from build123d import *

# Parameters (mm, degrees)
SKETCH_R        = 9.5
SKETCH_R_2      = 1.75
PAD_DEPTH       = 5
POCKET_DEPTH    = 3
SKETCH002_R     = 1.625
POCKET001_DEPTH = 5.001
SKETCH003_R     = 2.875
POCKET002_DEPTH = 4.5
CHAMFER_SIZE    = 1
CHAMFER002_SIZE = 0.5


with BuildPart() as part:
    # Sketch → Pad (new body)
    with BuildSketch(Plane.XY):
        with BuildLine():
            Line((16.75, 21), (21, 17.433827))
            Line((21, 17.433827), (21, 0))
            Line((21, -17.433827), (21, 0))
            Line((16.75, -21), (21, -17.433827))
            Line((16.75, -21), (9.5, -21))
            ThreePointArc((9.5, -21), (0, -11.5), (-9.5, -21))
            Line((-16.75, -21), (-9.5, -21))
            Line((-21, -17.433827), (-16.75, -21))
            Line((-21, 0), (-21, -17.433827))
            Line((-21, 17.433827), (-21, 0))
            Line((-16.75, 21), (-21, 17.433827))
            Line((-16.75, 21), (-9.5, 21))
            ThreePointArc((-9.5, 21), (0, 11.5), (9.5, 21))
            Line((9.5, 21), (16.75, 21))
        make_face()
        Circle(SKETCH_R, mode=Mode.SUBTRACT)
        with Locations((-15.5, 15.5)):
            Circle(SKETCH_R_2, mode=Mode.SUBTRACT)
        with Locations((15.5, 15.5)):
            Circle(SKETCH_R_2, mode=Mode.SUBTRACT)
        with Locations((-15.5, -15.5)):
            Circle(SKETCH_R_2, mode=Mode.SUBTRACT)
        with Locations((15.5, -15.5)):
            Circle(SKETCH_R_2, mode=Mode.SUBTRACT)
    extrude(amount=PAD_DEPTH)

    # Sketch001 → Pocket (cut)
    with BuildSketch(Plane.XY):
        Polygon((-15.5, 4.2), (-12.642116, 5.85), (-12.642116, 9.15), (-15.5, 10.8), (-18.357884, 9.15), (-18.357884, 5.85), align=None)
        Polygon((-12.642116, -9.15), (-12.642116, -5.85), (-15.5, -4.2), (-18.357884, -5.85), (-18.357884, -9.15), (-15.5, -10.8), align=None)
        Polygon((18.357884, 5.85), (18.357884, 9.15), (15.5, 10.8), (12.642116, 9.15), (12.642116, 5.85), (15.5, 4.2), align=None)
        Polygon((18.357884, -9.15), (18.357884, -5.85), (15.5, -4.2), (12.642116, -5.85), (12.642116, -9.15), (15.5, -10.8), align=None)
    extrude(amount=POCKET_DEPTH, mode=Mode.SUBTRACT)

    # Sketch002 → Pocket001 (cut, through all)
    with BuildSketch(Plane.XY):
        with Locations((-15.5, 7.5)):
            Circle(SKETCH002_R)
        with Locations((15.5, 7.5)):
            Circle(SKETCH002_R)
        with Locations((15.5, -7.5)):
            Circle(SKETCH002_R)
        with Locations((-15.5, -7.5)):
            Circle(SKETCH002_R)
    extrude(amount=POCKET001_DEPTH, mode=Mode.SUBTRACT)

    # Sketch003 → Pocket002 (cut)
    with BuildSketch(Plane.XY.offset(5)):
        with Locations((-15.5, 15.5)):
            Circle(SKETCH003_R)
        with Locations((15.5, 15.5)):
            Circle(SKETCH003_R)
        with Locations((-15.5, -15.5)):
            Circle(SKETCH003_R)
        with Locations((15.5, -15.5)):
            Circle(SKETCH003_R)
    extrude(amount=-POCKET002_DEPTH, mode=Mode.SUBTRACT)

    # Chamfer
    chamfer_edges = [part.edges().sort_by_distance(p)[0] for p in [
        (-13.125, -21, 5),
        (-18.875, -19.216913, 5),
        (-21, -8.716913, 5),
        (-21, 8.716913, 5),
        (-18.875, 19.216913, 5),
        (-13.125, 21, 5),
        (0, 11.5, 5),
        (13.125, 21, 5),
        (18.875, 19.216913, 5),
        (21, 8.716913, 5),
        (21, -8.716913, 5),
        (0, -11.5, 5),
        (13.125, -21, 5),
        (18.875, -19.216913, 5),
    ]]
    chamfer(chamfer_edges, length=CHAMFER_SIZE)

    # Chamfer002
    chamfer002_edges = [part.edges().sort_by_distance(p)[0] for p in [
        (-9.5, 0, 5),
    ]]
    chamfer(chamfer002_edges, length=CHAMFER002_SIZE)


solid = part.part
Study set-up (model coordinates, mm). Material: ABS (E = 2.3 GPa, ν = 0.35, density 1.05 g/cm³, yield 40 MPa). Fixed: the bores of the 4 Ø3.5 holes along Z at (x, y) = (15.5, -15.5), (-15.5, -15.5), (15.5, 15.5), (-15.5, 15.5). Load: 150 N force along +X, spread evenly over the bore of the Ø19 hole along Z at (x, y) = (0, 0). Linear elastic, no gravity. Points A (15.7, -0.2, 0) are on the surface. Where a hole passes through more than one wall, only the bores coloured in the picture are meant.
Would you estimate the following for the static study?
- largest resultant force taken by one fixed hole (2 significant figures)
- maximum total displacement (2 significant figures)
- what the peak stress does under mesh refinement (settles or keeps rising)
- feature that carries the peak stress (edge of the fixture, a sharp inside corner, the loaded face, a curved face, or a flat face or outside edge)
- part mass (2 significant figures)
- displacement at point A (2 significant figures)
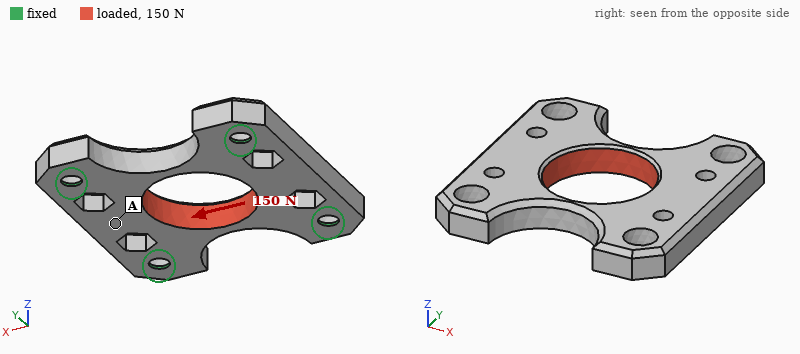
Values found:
39 N
35 µm
keeps rising
edge of the fixture
5.1 g
29 µm
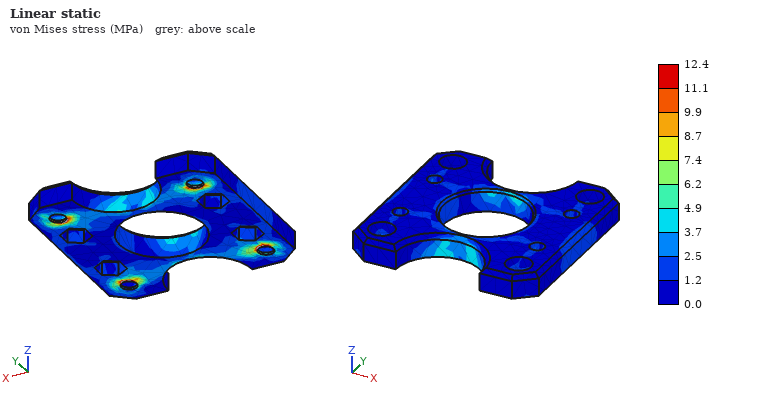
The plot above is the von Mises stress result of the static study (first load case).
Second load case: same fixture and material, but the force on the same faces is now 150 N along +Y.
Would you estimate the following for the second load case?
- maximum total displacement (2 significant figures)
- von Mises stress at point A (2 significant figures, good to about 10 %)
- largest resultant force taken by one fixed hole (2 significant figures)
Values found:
40 µm
1.5 MPa
41 N
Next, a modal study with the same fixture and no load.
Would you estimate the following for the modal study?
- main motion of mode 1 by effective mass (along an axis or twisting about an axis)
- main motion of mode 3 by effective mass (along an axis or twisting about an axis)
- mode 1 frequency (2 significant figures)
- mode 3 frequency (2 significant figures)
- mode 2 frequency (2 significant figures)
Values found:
along Z
along Z
3200 Hz
4300 Hz
3900 Hz
